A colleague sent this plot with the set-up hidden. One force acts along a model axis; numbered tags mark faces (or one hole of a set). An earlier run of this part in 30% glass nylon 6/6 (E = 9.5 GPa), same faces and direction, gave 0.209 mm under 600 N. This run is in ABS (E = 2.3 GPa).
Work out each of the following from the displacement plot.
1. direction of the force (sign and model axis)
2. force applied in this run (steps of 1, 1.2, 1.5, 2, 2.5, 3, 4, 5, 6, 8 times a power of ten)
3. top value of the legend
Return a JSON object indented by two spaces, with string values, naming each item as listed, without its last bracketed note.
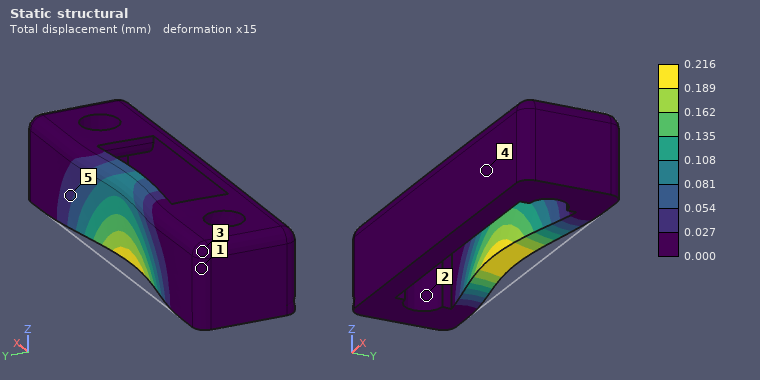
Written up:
{
  "direction of the force": "-Y",
  "force applied in this run": "150 N",
  "top value of the legend": "0.216 mm"
}
